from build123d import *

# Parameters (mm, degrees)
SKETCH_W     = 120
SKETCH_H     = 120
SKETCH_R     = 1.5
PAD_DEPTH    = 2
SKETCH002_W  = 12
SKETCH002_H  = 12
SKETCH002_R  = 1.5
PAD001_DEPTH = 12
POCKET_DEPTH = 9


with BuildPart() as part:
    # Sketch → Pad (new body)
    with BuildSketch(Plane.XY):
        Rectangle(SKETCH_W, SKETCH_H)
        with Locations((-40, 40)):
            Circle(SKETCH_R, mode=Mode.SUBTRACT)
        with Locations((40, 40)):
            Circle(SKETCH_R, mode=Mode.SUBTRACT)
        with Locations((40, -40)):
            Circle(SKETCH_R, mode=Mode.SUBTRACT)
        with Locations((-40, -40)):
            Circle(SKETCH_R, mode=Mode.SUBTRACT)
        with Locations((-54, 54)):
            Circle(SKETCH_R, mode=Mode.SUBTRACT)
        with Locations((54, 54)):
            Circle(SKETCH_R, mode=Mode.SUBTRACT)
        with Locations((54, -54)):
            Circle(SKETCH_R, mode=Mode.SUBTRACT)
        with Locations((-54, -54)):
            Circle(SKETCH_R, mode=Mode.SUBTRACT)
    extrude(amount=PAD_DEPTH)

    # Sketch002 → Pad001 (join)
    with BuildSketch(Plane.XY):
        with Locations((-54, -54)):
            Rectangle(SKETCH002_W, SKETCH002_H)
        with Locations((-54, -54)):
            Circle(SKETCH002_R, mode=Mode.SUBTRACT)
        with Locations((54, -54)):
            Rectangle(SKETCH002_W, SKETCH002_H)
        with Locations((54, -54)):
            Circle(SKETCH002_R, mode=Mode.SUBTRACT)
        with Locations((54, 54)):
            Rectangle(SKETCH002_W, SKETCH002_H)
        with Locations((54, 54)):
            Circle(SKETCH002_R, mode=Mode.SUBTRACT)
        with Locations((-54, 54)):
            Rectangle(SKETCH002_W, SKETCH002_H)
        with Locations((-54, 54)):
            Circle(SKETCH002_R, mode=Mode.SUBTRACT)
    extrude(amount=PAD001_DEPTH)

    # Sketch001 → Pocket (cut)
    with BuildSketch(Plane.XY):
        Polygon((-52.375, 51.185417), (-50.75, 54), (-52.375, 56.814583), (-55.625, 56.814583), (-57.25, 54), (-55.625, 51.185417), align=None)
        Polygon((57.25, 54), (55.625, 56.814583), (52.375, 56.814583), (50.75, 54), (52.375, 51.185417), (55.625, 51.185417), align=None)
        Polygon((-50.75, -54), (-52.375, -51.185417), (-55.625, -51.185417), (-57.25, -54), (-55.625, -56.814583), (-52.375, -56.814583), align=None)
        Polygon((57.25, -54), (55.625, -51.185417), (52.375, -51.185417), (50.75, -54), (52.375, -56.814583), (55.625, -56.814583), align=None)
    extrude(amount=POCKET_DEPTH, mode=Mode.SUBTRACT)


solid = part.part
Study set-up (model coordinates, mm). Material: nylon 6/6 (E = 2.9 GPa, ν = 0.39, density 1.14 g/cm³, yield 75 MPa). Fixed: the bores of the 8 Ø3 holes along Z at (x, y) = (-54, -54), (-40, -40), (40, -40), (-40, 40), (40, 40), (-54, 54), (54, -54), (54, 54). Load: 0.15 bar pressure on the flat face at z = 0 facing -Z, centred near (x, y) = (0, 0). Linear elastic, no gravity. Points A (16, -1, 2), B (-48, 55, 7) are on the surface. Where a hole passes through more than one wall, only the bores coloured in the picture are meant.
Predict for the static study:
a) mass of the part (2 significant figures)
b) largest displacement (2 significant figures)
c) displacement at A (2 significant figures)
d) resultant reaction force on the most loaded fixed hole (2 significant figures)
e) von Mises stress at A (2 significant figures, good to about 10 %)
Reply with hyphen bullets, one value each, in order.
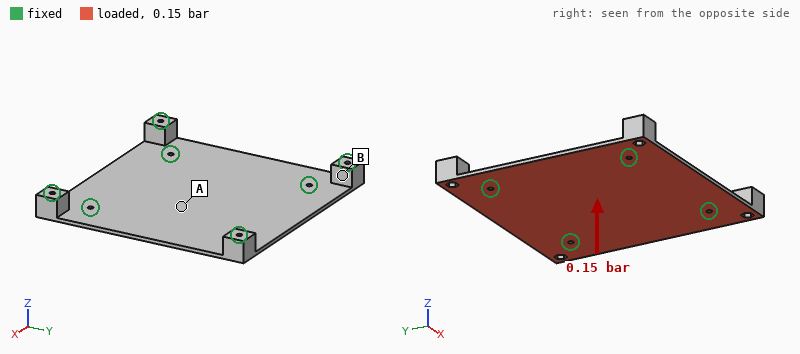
- 38 g
- 1.8 mm
- 1.7 mm
- 60 N
- 6.4 MPa
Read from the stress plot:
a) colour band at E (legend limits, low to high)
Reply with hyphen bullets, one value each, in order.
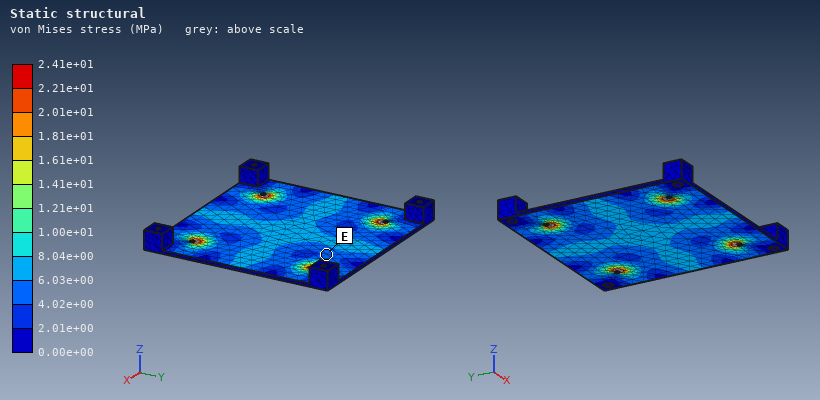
- 4.02e+00 to 6.03e+00 MPa
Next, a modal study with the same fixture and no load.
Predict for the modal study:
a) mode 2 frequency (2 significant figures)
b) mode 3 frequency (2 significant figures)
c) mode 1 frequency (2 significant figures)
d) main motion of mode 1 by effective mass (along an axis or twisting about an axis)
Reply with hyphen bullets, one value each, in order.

- 490 Hz
- 510 Hz
- 370 Hz
- along Z
